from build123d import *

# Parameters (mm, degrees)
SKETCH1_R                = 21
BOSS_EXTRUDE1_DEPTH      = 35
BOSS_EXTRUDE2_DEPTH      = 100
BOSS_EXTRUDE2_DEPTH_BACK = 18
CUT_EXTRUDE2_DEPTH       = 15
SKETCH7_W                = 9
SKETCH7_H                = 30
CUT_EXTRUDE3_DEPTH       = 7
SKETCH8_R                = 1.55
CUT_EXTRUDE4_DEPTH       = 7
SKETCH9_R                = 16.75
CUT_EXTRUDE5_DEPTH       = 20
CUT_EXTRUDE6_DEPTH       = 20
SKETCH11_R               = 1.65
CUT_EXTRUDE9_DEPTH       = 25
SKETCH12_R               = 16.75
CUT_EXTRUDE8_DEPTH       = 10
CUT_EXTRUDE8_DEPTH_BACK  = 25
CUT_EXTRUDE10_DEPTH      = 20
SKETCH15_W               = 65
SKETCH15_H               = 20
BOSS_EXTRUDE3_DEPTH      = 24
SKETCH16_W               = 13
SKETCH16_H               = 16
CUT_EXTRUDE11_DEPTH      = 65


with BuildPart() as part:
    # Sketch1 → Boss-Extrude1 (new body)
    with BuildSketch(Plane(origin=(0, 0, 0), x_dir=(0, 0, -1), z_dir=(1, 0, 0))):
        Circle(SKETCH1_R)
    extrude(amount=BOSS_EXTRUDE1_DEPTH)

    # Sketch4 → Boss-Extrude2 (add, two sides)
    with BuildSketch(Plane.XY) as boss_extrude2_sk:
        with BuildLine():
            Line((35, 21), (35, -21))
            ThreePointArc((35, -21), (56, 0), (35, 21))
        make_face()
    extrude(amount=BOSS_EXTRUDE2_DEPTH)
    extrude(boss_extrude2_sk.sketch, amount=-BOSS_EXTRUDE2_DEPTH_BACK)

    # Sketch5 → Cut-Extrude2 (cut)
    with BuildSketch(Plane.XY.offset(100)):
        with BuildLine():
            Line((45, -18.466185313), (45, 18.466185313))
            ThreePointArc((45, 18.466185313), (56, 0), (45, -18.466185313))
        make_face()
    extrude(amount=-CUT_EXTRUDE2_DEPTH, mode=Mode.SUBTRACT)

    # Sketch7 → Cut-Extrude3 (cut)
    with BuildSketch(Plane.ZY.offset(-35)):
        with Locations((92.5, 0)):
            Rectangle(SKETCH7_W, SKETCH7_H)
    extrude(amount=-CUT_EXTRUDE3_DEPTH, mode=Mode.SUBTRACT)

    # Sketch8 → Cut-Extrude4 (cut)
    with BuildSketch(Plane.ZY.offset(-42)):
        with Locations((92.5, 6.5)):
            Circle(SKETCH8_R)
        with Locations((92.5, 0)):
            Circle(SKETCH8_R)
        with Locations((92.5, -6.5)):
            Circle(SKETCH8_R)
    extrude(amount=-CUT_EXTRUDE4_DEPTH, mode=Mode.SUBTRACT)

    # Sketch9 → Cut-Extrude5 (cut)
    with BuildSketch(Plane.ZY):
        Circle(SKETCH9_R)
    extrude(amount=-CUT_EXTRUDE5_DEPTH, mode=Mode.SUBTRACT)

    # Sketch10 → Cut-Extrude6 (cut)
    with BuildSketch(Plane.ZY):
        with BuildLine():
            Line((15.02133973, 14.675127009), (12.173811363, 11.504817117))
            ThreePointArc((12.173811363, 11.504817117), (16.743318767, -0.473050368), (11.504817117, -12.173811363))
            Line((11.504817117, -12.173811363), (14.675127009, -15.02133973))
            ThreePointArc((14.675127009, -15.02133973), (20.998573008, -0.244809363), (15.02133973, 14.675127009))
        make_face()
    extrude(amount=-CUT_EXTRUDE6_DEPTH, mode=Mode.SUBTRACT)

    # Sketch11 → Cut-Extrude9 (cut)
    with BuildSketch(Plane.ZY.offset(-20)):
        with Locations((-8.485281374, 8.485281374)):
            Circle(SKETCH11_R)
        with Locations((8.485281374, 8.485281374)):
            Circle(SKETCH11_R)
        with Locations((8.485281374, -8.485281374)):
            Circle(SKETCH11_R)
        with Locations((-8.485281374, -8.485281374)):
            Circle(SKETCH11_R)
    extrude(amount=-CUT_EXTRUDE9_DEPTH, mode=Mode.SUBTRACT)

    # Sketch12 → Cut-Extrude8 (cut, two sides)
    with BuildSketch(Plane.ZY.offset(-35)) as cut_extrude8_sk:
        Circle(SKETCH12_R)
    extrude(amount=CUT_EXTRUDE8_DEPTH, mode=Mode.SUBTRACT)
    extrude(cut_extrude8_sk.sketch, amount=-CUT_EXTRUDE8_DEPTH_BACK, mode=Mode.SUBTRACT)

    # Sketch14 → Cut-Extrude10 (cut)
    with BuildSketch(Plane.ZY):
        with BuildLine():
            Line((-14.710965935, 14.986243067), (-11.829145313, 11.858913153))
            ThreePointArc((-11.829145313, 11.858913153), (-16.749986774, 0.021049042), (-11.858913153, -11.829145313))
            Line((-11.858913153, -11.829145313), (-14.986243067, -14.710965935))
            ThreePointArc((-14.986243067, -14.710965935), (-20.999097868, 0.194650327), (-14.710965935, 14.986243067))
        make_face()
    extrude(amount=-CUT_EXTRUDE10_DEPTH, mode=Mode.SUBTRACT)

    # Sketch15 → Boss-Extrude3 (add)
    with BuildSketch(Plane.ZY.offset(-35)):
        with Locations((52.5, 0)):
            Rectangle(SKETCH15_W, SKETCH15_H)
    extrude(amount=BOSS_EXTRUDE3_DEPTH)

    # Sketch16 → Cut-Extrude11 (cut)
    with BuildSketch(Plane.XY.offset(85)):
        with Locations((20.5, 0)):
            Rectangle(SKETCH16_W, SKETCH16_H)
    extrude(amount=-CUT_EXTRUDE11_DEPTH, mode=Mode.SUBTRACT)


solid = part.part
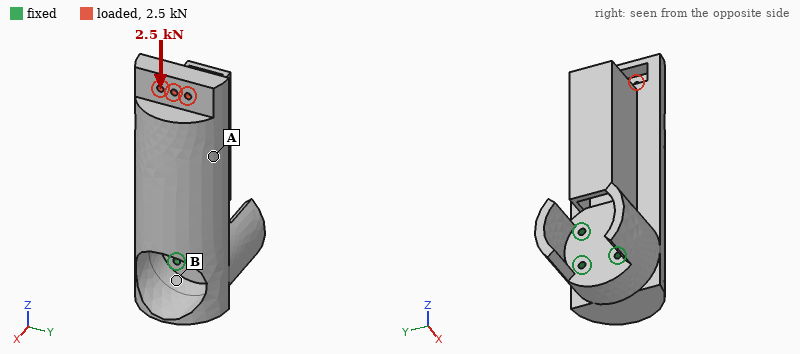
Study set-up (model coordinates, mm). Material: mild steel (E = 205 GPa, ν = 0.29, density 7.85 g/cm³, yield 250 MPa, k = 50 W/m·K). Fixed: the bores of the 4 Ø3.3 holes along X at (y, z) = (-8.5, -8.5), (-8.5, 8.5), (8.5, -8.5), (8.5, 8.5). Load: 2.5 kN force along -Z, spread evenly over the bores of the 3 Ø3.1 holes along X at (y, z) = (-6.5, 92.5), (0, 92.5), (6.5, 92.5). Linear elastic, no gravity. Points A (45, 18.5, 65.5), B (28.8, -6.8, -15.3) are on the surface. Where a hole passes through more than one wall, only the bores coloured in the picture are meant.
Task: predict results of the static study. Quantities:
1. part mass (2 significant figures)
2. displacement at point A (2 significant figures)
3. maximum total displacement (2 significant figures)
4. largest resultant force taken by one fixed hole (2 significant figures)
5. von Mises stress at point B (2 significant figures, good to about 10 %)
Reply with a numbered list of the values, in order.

1. 730 g
2. 33 µm
3. 53 µm
4. 1.3 kN
5. 17 MPa
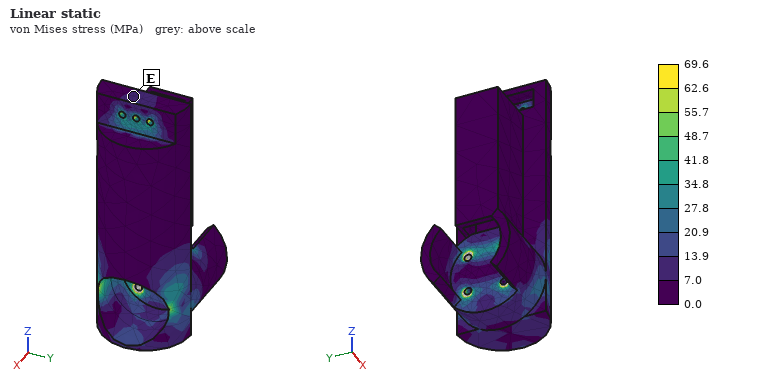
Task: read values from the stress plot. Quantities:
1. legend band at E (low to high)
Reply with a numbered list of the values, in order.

1. 7.0 to 13.9 MPa
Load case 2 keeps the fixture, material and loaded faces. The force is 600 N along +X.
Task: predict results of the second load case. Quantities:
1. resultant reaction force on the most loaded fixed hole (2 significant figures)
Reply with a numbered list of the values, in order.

1. 1.4 kN
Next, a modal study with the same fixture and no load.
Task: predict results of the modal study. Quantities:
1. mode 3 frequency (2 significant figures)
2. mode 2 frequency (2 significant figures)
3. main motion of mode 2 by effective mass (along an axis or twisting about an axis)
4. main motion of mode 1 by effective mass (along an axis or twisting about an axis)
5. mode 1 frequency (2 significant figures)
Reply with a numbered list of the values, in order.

1. 3600 Hz
2. 1700 Hz
3. along Y
4. along X
5. 1100 Hz
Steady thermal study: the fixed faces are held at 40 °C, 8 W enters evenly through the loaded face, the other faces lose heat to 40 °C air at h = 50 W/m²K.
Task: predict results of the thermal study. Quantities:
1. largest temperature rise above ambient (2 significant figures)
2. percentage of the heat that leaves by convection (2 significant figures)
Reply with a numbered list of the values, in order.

1. 22 K
2. 76 %
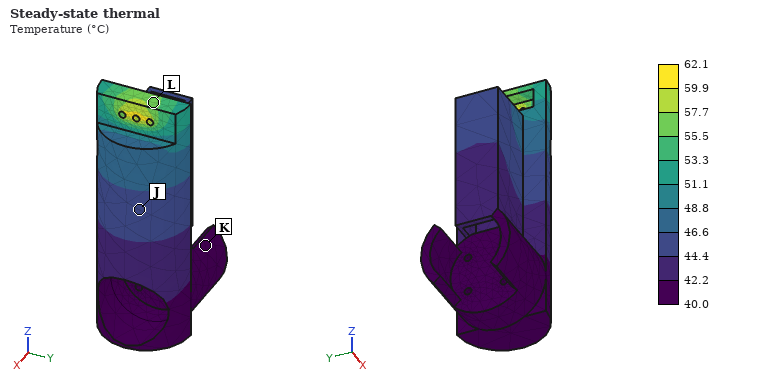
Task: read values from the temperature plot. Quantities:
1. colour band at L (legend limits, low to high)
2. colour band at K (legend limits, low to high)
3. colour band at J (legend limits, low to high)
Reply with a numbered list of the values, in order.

1. 55.5 to 57.7 °C
2. 40.0 to 42.2 °C
3. 44.4 to 46.6 °C
